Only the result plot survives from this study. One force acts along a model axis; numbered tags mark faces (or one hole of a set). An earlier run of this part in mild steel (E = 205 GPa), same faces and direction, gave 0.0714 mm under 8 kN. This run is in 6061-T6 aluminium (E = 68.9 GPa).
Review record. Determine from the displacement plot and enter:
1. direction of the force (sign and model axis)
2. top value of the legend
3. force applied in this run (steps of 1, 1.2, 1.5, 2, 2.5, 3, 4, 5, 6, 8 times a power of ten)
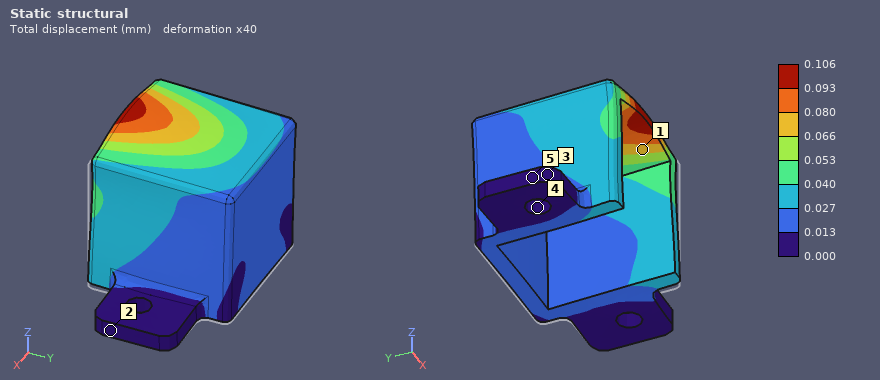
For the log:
+Z
0.106 mm
4 kN
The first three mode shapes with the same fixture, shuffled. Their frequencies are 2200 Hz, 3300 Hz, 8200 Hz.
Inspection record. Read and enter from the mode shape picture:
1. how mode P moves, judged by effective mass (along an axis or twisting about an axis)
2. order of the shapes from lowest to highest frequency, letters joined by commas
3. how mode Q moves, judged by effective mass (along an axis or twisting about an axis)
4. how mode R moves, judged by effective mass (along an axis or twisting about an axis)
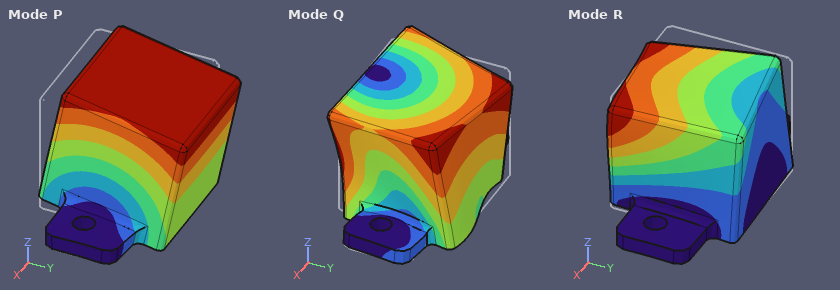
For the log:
along Y
P, R, Q
along X
along X
